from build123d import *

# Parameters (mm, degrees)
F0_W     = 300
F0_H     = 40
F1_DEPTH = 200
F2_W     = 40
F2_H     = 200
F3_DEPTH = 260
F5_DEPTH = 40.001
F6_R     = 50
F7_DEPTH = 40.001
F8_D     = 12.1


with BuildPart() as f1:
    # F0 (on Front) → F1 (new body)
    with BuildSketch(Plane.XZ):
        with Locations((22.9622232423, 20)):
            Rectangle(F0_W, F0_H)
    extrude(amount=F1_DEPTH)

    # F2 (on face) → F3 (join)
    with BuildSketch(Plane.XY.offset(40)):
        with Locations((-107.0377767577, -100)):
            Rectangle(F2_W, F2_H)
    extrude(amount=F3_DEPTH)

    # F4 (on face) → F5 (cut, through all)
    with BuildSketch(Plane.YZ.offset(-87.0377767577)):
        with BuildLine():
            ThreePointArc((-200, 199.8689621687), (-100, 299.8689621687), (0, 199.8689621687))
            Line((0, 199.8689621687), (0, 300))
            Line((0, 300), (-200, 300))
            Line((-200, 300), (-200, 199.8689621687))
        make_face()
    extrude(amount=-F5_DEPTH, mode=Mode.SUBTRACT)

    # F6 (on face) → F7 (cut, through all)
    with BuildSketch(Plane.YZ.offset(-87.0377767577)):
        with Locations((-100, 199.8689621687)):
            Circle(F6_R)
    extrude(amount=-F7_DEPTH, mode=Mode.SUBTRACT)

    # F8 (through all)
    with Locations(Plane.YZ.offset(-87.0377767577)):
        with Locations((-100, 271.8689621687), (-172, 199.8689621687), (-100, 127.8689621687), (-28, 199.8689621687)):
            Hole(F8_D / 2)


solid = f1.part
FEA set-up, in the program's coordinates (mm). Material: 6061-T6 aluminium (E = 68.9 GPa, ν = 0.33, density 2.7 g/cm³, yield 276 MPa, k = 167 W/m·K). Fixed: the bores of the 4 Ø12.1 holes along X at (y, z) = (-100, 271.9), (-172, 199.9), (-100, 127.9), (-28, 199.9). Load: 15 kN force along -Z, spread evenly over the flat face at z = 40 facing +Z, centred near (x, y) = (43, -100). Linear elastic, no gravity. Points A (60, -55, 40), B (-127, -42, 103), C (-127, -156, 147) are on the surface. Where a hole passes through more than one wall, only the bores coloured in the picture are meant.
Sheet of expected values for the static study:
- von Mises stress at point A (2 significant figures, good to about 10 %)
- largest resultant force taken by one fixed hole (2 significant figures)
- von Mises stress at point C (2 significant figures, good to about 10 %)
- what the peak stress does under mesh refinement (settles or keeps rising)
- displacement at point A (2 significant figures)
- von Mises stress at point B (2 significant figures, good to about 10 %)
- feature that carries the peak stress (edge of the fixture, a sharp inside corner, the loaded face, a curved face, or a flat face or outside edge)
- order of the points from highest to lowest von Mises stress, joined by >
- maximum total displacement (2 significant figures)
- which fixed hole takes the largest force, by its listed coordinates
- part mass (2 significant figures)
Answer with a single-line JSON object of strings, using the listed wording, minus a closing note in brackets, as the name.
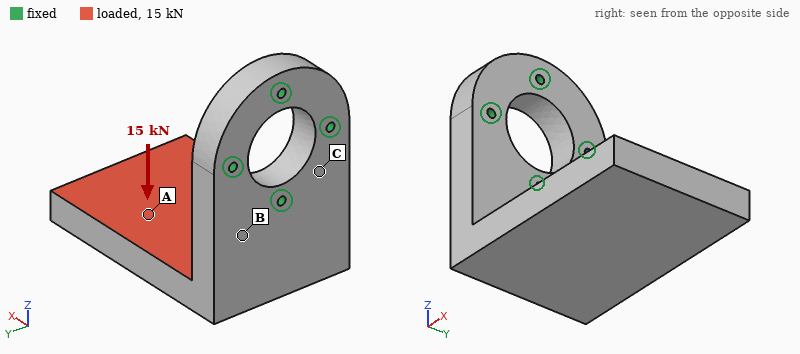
{"von Mises stress at point A": "7.2 MPa", "largest resultant force taken by one fixed hole": "18 kN", "von Mises stress at point C": "21 MPa", "what the peak stress does under mesh refinement": "keeps rising", "displacement at point A": "0.85 mm", "von Mises stress at point B": "33 MPa", "feature that carries the peak stress": "edge of the fixture", "order of the points from highest to lowest von Mises stress, joined by >": "B > C > A", "maximum total displacement": "1.6 mm", "which fixed hole takes the largest force, by its listed coordinates": "(-100, 127.9)", "part mass": "11 kg"}
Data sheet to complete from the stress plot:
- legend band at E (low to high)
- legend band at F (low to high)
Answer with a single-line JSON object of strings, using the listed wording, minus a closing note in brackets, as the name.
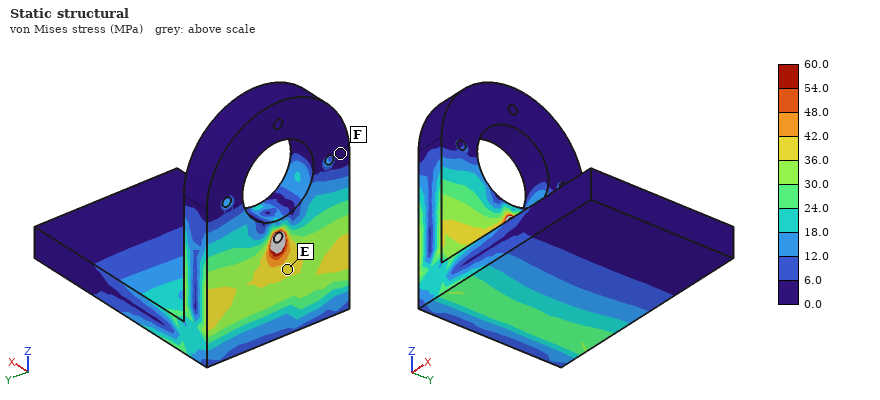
{"legend band at E": "36.0 to 42.0 MPa", "legend band at F": "0.0 to 6.0 MPa"}
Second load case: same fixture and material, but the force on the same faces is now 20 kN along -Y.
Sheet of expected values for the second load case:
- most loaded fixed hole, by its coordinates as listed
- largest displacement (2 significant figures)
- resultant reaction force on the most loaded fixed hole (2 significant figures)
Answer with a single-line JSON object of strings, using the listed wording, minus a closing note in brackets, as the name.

{"most loaded fixed hole, by its coordinates as listed": "(-100, 127.9)", "largest displacement": "1.1 mm", "resultant reaction force on the most loaded fixed hole": "20 kN"}
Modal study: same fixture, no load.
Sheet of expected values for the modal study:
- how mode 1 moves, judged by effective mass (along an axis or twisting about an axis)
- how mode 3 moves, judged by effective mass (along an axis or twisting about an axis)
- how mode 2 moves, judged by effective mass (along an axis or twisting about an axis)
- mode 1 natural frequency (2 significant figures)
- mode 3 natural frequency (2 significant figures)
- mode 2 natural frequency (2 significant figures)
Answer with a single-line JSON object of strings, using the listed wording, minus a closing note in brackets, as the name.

{"how mode 1 moves, judged by effective mass": "along Z", "how mode 3 moves, judged by effective mass": "along X", "how mode 2 moves, judged by effective mass": "along Y", "mode 1 natural frequency": "250 Hz", "mode 3 natural frequency": "830 Hz", "mode 2 natural frequency": "350 Hz"}
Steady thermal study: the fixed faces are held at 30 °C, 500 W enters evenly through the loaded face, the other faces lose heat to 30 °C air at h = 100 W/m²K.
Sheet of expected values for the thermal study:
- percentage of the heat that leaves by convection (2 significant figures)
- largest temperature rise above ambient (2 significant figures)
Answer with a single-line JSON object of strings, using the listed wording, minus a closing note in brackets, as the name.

{"percentage of the heat that leaves by convection": "69 %", "largest temperature rise above ambient": "39 K"}
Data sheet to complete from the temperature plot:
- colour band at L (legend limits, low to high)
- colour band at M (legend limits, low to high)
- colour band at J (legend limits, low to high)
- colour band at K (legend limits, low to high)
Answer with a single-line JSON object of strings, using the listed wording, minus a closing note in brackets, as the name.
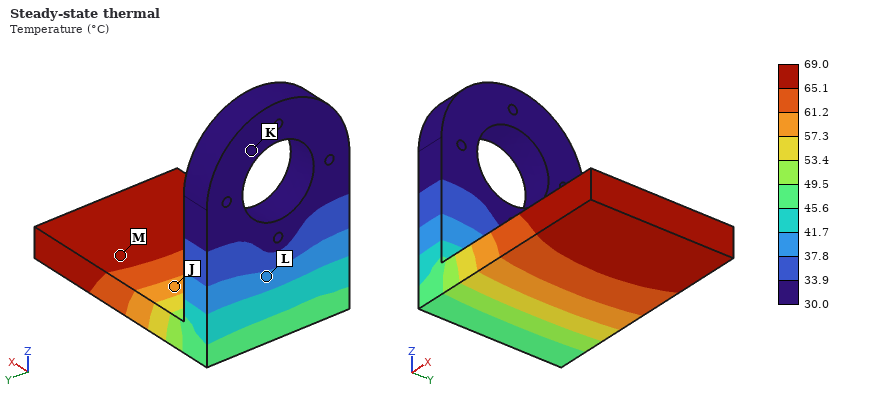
{"colour band at L": "37.8 to 41.7 °C", "colour band at M": "65.1 to 69.0 °C", "colour band at J": "57.3 to 61.2 °C", "colour band at K": "30.0 to 33.9 °C"}
